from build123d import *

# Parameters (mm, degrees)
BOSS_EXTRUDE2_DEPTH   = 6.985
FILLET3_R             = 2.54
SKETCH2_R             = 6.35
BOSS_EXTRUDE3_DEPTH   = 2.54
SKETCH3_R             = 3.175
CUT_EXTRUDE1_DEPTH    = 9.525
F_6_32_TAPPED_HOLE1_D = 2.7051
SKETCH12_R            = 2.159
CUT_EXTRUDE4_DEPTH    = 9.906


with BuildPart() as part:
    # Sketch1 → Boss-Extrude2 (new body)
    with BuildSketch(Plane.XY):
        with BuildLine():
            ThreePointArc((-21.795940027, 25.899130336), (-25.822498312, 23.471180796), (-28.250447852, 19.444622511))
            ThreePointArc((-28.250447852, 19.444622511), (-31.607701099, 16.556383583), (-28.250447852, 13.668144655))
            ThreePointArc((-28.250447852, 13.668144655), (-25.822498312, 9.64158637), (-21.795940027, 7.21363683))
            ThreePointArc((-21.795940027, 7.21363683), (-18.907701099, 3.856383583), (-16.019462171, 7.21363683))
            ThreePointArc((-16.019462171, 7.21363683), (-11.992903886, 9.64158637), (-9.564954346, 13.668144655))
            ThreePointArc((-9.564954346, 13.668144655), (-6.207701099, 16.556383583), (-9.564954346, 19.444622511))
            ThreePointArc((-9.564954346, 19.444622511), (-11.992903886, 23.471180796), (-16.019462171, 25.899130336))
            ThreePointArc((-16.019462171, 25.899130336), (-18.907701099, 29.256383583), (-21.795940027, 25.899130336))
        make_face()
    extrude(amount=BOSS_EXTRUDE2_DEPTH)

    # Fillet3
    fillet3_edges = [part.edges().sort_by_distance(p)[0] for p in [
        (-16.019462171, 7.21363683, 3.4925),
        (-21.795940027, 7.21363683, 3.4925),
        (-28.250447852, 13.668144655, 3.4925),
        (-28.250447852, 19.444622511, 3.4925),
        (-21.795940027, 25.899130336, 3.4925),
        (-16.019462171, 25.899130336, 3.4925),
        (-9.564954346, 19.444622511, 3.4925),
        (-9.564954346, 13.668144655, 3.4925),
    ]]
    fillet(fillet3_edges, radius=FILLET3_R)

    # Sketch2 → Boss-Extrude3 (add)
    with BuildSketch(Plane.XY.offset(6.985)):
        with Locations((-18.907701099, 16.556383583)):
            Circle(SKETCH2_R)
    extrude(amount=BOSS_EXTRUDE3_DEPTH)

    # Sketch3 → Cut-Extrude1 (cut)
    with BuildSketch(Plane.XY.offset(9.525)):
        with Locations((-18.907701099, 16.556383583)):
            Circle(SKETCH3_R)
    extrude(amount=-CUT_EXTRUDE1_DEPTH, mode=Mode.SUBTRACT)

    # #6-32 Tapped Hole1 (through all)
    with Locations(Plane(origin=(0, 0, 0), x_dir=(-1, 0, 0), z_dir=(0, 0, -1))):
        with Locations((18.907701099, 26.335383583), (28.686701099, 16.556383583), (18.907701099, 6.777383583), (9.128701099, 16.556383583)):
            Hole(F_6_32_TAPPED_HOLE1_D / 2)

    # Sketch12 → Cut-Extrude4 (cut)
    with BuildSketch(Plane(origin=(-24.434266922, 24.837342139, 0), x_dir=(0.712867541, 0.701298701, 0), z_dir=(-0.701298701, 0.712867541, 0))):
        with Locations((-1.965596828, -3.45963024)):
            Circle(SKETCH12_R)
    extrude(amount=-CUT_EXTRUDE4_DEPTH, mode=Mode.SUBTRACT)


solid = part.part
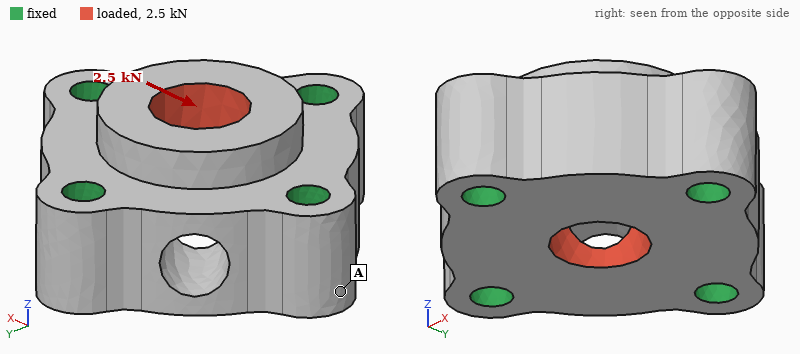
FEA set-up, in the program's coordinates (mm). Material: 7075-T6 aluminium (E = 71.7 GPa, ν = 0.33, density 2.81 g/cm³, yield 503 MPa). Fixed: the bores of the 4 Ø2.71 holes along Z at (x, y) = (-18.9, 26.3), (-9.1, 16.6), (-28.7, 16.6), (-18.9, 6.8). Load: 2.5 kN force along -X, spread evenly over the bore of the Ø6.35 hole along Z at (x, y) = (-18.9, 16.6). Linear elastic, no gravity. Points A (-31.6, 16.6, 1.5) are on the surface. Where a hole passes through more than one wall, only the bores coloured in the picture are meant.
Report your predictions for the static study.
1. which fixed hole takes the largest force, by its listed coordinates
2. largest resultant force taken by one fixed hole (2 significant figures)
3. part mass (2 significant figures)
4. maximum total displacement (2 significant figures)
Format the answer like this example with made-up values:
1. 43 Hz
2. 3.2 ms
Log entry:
1. (-9.1, 16.6)
2. 980 N
3. 6.4 g
4. 3.5 µm
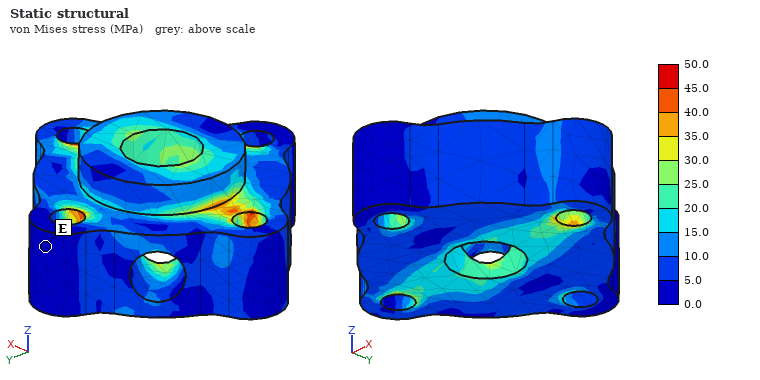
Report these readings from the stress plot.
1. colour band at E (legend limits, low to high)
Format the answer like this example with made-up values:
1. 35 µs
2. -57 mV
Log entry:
1. 0.0 to 5.0 MPa
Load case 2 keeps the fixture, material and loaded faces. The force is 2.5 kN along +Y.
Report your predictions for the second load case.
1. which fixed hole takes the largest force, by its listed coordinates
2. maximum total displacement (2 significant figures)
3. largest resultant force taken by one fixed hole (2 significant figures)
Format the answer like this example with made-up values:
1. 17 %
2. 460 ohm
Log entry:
1. (-18.9, 6.8)
2. 3.5 µm
3. 980 N
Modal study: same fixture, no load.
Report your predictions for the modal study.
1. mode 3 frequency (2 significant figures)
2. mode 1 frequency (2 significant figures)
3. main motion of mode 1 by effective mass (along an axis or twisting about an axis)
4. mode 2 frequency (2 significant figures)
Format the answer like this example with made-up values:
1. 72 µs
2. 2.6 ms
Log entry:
1. 95 kHz
2. 84 kHz
3. along Z
4. 92 kHz
